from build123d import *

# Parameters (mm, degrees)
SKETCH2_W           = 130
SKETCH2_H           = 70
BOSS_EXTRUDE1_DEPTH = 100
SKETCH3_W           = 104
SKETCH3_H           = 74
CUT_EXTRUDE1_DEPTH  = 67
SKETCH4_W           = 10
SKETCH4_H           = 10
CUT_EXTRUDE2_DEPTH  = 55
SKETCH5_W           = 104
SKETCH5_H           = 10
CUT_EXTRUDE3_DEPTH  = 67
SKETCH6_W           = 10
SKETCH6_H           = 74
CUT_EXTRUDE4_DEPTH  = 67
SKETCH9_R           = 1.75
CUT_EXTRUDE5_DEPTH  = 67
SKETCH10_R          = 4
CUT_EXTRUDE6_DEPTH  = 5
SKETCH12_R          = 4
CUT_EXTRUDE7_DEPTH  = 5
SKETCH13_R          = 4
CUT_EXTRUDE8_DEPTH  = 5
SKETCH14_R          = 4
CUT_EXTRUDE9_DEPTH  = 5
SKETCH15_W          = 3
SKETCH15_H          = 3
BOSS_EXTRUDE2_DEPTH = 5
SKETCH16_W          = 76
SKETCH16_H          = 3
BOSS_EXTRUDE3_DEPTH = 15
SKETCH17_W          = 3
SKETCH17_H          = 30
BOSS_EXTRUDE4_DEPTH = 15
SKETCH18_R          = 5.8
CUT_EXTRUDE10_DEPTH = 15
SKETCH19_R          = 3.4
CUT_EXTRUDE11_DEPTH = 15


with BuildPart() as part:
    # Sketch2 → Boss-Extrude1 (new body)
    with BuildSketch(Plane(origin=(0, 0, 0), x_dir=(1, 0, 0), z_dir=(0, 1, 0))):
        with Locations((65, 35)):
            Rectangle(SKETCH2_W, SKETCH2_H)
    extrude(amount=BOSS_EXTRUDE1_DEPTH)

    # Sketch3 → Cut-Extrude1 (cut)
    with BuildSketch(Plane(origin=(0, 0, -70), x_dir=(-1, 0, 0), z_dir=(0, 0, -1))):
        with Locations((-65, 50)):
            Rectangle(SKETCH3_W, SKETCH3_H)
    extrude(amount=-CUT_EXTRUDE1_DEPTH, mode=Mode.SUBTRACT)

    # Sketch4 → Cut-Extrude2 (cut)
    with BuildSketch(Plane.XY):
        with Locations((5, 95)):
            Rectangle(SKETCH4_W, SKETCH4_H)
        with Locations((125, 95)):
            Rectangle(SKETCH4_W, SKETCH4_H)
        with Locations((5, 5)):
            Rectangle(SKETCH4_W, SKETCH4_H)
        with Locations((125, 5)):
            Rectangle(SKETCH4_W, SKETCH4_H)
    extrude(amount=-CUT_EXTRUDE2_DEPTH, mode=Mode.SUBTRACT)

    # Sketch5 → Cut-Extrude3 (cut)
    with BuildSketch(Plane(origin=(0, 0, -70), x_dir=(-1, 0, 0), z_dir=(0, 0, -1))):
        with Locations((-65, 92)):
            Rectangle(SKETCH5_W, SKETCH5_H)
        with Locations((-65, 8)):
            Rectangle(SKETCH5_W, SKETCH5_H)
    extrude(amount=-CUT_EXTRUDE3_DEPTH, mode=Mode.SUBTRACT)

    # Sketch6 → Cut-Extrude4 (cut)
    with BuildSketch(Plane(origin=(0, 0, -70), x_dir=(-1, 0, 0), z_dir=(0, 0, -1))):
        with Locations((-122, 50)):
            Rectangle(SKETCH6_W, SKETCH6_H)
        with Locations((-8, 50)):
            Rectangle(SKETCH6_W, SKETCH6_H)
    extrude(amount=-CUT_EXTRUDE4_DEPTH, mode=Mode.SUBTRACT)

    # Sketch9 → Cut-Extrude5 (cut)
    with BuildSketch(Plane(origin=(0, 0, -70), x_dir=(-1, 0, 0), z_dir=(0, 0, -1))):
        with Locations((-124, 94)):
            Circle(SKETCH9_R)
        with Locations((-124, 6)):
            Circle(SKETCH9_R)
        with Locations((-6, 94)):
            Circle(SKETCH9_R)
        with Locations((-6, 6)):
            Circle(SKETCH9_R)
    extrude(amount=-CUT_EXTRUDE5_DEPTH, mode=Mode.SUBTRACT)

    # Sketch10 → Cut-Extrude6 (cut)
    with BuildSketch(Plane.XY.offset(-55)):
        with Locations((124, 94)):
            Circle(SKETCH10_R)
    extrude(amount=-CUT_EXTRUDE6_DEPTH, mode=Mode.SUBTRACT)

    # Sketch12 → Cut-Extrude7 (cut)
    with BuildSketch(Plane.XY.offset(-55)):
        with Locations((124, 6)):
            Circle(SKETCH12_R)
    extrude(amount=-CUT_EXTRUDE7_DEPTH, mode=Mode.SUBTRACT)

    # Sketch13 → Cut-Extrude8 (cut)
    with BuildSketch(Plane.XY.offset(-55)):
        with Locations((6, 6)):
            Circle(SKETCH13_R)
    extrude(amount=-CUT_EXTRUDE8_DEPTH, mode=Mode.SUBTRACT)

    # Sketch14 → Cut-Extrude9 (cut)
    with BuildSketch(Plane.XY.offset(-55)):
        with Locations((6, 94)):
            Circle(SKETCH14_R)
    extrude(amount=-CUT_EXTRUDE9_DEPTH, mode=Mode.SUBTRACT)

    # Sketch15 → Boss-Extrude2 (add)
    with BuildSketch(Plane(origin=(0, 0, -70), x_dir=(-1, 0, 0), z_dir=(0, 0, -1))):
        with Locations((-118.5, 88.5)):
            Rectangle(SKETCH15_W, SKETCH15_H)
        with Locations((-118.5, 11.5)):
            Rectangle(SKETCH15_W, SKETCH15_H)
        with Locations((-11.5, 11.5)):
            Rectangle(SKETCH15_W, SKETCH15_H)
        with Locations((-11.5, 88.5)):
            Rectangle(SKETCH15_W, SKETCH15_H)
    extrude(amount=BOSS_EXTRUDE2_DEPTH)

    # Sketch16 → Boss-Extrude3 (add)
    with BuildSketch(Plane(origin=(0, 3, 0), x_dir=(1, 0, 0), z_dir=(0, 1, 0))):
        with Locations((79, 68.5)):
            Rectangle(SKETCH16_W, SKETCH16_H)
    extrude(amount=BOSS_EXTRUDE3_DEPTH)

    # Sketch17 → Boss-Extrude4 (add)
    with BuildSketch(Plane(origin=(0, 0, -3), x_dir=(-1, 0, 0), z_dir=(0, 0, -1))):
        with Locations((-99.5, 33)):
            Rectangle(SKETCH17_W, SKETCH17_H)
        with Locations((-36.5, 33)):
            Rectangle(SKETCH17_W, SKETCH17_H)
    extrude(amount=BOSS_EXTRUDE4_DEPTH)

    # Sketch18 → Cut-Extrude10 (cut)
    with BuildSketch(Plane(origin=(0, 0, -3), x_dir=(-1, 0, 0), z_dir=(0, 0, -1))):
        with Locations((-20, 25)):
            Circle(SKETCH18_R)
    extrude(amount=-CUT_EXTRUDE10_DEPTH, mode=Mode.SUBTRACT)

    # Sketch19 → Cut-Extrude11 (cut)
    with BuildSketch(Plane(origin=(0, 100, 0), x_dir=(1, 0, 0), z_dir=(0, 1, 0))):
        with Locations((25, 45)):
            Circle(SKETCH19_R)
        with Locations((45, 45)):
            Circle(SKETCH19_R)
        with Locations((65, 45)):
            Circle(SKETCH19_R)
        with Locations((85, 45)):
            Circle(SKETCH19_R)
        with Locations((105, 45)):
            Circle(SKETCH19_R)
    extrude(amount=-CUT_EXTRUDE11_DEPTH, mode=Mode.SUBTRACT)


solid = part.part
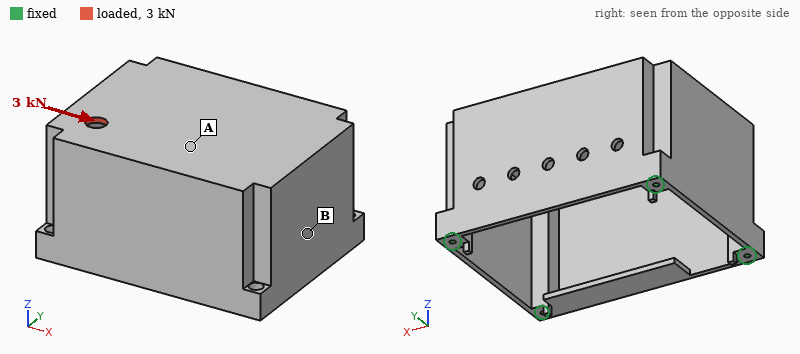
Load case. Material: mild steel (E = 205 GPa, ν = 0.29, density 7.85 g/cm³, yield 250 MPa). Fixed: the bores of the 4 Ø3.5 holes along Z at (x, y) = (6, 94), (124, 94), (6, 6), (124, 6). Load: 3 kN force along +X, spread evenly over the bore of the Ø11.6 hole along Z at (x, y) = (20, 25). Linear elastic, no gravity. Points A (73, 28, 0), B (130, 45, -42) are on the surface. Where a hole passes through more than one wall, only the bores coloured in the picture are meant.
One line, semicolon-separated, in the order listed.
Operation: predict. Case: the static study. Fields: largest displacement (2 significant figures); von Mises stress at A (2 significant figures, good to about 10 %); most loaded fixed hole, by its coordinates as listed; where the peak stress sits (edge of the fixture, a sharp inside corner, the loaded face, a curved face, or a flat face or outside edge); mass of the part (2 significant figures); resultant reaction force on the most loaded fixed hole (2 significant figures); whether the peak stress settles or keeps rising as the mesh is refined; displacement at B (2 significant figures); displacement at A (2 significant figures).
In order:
12 µm; 7.4 MPa; (124, 6); a sharp inside corner; 1.1 kg; 1.4 kN; keeps rising; 2.1 µm; 7.0 µm
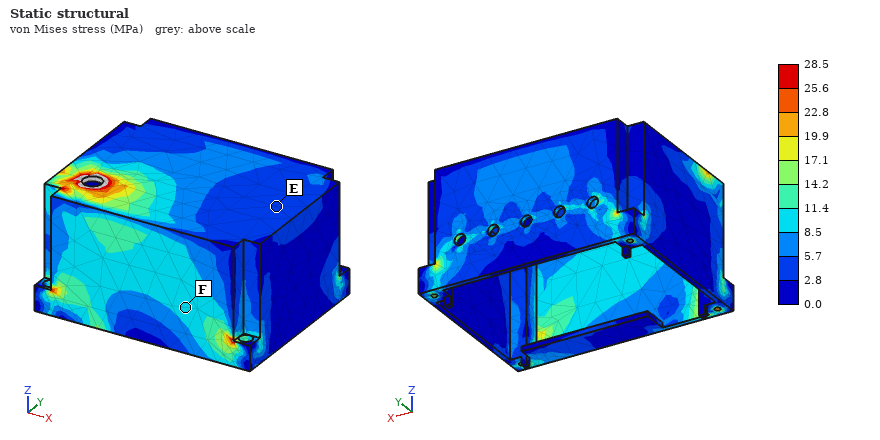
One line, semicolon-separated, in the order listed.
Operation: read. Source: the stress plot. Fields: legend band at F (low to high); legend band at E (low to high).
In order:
8.5 to 11.4 MPa; 2.8 to 5.7 MPa
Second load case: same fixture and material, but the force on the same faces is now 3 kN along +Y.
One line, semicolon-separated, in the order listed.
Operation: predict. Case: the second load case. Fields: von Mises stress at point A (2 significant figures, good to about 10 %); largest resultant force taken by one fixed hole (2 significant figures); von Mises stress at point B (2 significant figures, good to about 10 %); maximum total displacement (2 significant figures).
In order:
5.2 MPa; 1.7 kN; 5.6 MPa; 14 µm
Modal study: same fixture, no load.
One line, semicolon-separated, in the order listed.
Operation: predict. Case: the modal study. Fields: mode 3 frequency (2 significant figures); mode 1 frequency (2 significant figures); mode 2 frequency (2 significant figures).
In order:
2200 Hz; 1500 Hz; 1800 Hz
